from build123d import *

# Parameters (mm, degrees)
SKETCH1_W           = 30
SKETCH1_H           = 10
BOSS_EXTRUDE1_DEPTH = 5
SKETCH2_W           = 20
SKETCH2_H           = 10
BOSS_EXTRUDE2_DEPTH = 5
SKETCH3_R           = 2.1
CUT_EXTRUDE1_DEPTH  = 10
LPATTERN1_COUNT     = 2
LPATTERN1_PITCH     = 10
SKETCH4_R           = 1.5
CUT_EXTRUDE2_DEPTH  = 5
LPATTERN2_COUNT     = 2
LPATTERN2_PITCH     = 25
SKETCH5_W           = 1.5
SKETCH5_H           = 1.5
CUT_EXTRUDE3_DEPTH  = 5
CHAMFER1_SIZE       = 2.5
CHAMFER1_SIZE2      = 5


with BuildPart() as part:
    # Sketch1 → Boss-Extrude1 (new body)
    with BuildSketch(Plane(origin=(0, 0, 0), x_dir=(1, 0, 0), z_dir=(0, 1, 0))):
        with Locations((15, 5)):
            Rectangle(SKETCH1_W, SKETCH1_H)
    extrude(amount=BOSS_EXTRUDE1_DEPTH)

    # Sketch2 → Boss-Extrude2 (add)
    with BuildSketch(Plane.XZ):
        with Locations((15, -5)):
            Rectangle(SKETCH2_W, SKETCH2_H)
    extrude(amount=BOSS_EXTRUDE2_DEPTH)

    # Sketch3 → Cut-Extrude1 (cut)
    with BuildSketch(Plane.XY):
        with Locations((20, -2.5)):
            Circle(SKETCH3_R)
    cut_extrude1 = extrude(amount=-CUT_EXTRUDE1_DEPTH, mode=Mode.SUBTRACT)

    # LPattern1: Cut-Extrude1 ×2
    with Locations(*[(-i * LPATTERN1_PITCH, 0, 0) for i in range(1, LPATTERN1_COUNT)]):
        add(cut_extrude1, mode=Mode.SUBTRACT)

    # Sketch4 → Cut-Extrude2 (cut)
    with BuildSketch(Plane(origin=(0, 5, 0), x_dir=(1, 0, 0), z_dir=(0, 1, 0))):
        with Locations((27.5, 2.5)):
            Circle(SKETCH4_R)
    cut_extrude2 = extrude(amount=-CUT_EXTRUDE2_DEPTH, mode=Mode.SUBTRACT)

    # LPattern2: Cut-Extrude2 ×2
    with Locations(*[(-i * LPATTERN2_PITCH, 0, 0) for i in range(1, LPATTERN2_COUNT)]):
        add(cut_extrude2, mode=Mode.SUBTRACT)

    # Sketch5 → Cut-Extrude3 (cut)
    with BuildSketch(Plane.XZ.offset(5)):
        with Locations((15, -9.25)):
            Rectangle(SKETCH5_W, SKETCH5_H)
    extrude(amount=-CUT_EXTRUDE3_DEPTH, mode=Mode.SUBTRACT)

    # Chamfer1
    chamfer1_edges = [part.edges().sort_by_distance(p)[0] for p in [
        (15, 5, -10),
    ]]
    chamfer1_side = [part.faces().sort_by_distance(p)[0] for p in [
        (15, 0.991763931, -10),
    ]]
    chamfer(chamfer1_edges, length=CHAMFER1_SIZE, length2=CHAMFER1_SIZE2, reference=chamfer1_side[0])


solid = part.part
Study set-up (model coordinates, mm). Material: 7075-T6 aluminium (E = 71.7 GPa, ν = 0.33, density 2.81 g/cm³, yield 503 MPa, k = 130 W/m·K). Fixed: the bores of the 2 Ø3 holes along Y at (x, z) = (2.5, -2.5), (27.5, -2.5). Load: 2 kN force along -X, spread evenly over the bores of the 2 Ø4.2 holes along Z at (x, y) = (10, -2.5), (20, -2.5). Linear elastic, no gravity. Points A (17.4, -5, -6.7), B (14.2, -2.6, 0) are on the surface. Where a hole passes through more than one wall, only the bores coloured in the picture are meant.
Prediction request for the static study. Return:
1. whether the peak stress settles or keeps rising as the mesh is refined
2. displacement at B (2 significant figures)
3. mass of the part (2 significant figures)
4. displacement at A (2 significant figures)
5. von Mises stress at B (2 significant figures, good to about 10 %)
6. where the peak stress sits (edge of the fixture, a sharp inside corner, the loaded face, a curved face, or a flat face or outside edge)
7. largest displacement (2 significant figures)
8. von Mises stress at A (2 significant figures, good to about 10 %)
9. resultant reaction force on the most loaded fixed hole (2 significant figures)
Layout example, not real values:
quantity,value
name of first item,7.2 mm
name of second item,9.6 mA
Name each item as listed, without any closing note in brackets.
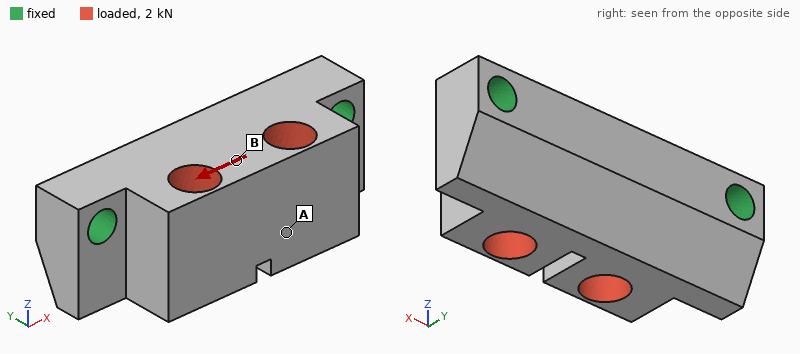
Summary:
quantity,value
whether the peak stress settles or keeps rising as the mesh is refined,keeps rising
displacement at B,5.6 µm
mass of the part,5.5 g
displacement at A,7.5 µm
von Mises stress at B,25 MPa
where the peak stress sits,a sharp inside corner
largest displacement,8.5 µm
von Mises stress at A,10 MPa
resultant reaction force on the most loaded fixed hole,1.1 kN
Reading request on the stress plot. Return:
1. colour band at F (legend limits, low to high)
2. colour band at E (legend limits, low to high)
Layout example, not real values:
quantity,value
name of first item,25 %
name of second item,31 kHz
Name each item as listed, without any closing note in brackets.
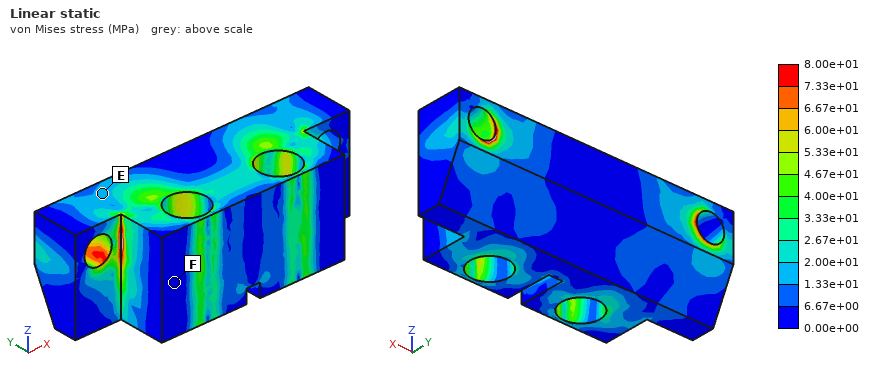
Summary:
quantity,value
colour band at F,0.00e+00 to 6.67e+00 MPa
colour band at E,1.33e+01 to 2.00e+01 MPa
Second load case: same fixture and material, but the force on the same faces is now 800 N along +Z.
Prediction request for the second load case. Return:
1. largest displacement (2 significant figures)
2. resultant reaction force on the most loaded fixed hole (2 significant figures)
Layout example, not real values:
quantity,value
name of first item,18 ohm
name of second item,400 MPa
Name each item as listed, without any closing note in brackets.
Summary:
quantity,value
largest displacement,19 µm
resultant reaction force on the most loaded fixed hole,440 N
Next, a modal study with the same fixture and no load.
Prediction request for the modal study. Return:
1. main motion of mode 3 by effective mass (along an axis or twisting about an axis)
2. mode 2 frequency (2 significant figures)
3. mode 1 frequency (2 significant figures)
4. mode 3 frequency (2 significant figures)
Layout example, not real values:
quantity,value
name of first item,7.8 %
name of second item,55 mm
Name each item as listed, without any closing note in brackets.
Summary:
quantity,value
main motion of mode 3 by effective mass,along Z
mode 2 frequency,34 kHz
mode 1 frequency,23 kHz
mode 3 frequency,42 kHz
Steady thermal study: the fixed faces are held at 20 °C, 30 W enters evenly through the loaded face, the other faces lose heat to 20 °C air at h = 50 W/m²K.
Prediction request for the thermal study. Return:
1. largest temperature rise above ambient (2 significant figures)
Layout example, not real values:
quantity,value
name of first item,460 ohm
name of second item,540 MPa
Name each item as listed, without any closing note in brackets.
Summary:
quantity,value
largest temperature rise above ambient,23 K
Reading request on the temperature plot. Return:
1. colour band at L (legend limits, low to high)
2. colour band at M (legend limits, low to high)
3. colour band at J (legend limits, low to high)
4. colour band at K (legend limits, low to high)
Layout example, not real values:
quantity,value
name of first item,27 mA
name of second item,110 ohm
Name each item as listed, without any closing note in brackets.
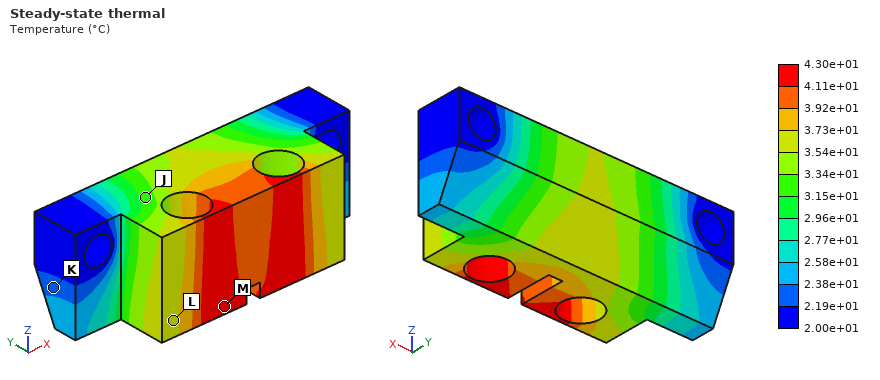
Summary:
quantity,value
colour band at L,3.54e+01 to 3.73e+01 °C
colour band at M,4.11e+01 to 4.30e+01 °C
colour band at J,3.15e+01 to 3.34e+01 °C
colour band at K,2.19e+01 to 2.38e+01 °C
